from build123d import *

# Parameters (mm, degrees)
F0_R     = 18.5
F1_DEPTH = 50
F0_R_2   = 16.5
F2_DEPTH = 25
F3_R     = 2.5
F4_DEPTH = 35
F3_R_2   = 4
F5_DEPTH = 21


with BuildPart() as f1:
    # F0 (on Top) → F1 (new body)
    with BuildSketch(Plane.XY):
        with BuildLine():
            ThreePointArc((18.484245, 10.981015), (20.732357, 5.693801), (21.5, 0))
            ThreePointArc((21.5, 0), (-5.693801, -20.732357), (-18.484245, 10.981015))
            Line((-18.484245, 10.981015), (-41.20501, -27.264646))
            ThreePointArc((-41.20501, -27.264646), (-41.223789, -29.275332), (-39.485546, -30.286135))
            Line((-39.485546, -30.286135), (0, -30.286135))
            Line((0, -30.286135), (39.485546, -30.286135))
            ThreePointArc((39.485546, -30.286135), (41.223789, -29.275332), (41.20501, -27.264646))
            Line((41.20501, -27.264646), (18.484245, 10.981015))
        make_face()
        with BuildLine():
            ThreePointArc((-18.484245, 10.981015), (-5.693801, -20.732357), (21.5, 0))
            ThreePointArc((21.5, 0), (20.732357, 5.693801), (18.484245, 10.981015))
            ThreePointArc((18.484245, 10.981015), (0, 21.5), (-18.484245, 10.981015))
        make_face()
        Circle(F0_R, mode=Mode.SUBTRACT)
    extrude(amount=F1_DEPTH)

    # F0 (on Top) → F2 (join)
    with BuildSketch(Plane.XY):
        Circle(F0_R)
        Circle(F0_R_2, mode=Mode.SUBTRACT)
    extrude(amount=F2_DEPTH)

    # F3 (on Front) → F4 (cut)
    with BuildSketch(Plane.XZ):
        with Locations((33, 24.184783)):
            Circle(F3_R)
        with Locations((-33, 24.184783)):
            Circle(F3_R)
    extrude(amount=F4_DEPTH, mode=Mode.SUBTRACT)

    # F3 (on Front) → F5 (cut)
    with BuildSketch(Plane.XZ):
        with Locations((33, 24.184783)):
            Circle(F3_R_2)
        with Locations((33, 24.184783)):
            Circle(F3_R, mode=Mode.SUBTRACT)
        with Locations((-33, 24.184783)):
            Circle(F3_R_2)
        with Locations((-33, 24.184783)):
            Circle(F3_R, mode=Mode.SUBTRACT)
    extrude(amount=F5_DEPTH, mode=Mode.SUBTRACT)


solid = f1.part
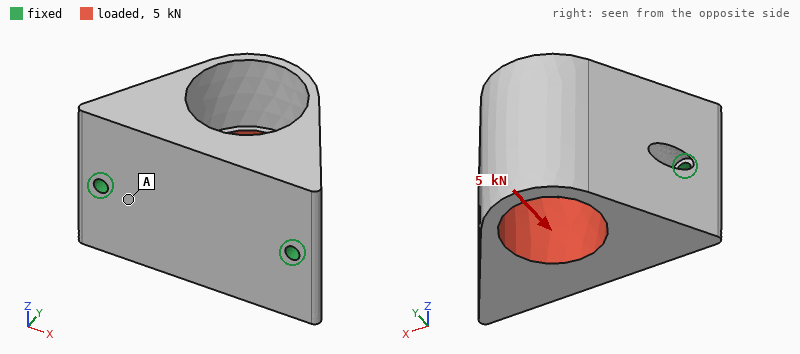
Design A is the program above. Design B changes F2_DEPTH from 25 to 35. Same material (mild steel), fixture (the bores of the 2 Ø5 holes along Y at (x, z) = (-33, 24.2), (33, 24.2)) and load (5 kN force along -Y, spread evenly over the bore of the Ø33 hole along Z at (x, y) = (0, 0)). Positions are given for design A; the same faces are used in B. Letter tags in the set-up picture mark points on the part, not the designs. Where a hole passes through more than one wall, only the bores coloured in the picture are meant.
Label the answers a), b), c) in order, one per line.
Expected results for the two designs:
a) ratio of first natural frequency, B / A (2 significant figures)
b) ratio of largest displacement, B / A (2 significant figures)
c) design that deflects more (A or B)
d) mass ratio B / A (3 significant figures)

a) 0.98
b) 0.59
c) A
d) 1.02
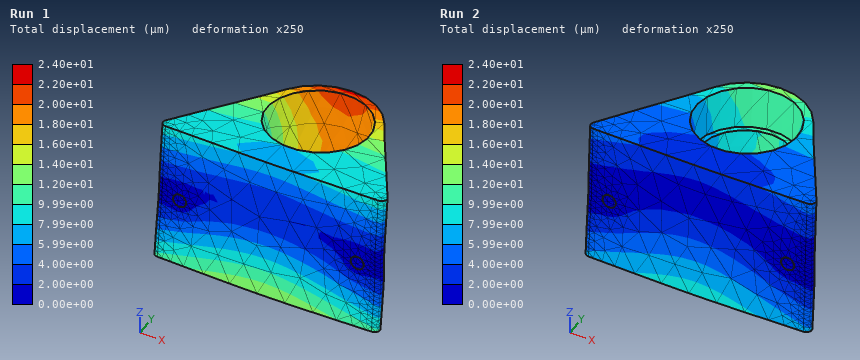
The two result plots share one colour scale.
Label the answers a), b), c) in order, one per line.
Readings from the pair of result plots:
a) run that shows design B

a) Run 2
